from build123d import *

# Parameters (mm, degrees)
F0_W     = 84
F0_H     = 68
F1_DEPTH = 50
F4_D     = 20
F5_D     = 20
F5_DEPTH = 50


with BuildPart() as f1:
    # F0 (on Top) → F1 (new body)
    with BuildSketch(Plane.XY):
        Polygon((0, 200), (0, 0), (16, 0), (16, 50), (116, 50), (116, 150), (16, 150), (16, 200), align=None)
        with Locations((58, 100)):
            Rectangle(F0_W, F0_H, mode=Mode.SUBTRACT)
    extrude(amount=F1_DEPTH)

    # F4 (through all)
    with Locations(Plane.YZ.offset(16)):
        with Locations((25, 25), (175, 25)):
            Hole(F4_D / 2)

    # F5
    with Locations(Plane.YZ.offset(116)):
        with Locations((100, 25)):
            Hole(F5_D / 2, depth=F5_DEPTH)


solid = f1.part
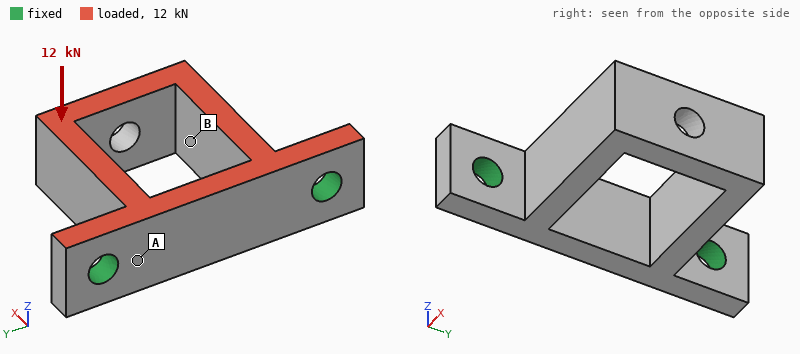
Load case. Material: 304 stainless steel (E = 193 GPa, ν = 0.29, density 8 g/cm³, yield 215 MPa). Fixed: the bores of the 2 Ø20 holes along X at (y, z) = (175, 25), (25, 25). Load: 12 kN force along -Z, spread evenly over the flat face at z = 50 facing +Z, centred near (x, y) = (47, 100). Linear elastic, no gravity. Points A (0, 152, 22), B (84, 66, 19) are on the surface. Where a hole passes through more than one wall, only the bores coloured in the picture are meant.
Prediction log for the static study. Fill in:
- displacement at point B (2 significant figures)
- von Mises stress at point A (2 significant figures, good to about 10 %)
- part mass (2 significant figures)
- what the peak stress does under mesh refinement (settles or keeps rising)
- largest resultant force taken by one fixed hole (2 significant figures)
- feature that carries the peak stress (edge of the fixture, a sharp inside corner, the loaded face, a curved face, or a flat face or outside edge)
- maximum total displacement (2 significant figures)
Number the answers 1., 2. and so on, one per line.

1. 0.093 mm
2. 45 MPa
3. 2.9 kg
4. keeps rising
5. 6.0 kN
6. edge of the fixture
7. 0.14 mm
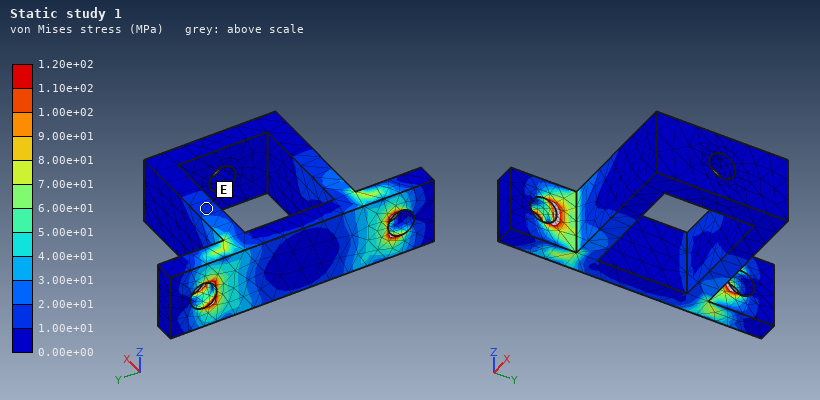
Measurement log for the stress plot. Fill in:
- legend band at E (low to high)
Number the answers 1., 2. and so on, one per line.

1. 1.00e+01 to 2.00e+01 MPa
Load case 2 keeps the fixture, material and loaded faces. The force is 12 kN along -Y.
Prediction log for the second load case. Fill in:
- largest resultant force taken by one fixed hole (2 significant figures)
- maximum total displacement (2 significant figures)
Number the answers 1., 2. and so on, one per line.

1. 7.2 kN
2. 94 µm
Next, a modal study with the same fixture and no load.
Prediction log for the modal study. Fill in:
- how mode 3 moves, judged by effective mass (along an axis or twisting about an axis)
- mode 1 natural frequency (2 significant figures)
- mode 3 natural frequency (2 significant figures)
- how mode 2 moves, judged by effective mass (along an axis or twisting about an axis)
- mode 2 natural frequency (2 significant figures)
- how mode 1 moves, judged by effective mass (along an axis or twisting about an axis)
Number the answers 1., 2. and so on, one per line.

1. twisting about X
2. 1000 Hz
3. 2100 Hz
4. along Y
5. 1300 Hz
6. along Z
